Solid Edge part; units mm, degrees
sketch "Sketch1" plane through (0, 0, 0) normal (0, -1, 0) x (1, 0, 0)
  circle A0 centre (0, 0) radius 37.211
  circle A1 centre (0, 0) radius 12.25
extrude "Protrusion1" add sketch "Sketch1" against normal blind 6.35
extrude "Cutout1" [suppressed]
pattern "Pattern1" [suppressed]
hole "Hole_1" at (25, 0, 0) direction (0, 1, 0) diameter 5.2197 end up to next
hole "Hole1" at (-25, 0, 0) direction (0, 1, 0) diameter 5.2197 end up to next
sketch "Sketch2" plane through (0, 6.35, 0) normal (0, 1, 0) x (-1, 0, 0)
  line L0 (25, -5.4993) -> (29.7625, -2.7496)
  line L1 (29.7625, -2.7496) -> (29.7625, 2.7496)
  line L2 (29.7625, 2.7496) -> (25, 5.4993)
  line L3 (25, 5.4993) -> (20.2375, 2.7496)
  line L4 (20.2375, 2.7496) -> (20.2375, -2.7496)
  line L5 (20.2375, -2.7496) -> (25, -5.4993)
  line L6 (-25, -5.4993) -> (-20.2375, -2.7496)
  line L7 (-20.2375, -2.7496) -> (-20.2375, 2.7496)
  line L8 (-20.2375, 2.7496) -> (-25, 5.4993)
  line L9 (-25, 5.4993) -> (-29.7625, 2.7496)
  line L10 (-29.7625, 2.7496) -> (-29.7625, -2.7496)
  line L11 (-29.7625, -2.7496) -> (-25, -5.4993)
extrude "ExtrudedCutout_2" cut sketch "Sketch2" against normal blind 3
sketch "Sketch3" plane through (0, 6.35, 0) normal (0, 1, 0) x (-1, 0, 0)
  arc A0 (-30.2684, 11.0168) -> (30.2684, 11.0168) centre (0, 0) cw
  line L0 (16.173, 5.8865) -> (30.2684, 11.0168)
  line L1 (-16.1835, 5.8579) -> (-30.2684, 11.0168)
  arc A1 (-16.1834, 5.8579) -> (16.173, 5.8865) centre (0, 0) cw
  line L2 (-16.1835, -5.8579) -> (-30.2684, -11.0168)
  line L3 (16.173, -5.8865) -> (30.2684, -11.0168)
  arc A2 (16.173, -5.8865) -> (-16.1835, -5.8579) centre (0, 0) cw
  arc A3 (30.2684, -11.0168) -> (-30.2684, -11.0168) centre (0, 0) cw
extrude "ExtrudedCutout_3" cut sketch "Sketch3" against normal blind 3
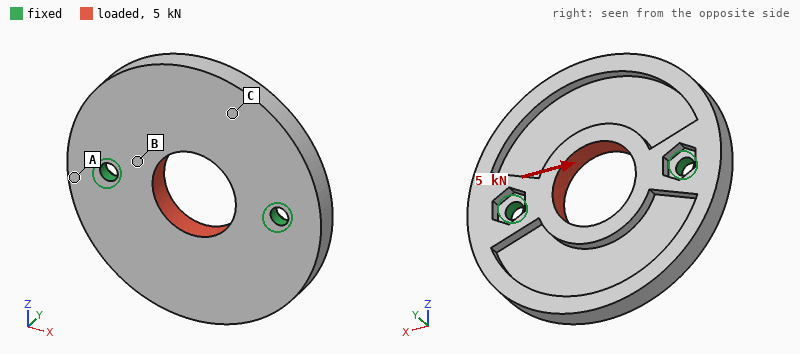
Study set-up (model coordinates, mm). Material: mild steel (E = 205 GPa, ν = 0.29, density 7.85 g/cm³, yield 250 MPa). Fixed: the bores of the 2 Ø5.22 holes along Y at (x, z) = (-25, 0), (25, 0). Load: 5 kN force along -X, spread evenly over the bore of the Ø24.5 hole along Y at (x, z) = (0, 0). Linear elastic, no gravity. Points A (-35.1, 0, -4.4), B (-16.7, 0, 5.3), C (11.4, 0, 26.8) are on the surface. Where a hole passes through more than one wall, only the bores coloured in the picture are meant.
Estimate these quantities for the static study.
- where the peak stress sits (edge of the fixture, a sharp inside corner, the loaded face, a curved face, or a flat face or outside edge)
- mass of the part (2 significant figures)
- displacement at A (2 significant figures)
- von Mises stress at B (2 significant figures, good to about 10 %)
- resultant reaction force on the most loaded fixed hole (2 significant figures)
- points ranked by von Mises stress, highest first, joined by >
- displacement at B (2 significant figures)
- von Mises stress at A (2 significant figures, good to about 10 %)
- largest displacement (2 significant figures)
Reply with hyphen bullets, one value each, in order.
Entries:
- edge of the fixture
- 150 g
- 1.1 µm
- 27 MPa
- 2.5 kN
- B > A > C
- 1.4 µm
- 14 MPa
- 3.6 µm
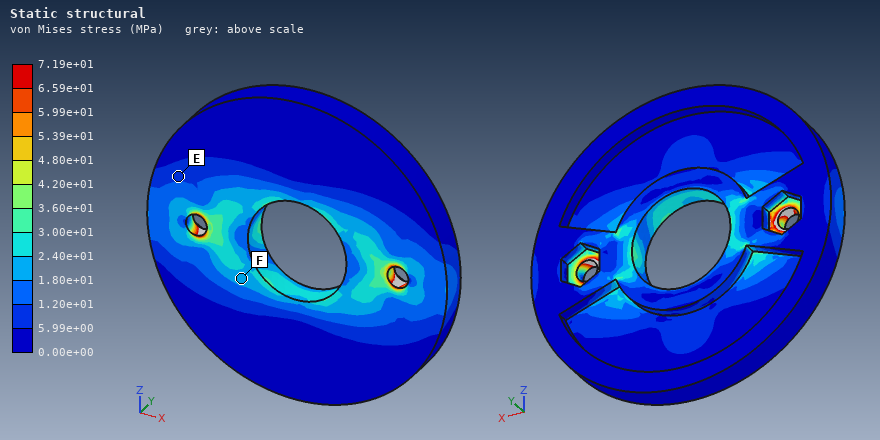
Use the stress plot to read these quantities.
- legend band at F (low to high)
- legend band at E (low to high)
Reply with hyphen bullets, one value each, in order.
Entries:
- 1.80e+01 to 2.40e+01 MPa
- 5.99e+00 to 1.20e+01 MPa
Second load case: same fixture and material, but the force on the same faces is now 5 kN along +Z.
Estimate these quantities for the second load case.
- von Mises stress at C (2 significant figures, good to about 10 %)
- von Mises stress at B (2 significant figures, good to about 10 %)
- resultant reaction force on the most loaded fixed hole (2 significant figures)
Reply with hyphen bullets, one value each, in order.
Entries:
- 12 MPa
- 23 MPa
- 2.5 kN
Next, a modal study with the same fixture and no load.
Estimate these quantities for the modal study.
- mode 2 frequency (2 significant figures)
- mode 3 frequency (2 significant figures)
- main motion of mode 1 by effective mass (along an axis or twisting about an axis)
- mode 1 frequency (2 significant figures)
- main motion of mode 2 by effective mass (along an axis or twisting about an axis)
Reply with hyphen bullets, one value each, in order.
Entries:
- 3300 Hz
- 6000 Hz
- twisting about X
- 2400 Hz
- along Y
